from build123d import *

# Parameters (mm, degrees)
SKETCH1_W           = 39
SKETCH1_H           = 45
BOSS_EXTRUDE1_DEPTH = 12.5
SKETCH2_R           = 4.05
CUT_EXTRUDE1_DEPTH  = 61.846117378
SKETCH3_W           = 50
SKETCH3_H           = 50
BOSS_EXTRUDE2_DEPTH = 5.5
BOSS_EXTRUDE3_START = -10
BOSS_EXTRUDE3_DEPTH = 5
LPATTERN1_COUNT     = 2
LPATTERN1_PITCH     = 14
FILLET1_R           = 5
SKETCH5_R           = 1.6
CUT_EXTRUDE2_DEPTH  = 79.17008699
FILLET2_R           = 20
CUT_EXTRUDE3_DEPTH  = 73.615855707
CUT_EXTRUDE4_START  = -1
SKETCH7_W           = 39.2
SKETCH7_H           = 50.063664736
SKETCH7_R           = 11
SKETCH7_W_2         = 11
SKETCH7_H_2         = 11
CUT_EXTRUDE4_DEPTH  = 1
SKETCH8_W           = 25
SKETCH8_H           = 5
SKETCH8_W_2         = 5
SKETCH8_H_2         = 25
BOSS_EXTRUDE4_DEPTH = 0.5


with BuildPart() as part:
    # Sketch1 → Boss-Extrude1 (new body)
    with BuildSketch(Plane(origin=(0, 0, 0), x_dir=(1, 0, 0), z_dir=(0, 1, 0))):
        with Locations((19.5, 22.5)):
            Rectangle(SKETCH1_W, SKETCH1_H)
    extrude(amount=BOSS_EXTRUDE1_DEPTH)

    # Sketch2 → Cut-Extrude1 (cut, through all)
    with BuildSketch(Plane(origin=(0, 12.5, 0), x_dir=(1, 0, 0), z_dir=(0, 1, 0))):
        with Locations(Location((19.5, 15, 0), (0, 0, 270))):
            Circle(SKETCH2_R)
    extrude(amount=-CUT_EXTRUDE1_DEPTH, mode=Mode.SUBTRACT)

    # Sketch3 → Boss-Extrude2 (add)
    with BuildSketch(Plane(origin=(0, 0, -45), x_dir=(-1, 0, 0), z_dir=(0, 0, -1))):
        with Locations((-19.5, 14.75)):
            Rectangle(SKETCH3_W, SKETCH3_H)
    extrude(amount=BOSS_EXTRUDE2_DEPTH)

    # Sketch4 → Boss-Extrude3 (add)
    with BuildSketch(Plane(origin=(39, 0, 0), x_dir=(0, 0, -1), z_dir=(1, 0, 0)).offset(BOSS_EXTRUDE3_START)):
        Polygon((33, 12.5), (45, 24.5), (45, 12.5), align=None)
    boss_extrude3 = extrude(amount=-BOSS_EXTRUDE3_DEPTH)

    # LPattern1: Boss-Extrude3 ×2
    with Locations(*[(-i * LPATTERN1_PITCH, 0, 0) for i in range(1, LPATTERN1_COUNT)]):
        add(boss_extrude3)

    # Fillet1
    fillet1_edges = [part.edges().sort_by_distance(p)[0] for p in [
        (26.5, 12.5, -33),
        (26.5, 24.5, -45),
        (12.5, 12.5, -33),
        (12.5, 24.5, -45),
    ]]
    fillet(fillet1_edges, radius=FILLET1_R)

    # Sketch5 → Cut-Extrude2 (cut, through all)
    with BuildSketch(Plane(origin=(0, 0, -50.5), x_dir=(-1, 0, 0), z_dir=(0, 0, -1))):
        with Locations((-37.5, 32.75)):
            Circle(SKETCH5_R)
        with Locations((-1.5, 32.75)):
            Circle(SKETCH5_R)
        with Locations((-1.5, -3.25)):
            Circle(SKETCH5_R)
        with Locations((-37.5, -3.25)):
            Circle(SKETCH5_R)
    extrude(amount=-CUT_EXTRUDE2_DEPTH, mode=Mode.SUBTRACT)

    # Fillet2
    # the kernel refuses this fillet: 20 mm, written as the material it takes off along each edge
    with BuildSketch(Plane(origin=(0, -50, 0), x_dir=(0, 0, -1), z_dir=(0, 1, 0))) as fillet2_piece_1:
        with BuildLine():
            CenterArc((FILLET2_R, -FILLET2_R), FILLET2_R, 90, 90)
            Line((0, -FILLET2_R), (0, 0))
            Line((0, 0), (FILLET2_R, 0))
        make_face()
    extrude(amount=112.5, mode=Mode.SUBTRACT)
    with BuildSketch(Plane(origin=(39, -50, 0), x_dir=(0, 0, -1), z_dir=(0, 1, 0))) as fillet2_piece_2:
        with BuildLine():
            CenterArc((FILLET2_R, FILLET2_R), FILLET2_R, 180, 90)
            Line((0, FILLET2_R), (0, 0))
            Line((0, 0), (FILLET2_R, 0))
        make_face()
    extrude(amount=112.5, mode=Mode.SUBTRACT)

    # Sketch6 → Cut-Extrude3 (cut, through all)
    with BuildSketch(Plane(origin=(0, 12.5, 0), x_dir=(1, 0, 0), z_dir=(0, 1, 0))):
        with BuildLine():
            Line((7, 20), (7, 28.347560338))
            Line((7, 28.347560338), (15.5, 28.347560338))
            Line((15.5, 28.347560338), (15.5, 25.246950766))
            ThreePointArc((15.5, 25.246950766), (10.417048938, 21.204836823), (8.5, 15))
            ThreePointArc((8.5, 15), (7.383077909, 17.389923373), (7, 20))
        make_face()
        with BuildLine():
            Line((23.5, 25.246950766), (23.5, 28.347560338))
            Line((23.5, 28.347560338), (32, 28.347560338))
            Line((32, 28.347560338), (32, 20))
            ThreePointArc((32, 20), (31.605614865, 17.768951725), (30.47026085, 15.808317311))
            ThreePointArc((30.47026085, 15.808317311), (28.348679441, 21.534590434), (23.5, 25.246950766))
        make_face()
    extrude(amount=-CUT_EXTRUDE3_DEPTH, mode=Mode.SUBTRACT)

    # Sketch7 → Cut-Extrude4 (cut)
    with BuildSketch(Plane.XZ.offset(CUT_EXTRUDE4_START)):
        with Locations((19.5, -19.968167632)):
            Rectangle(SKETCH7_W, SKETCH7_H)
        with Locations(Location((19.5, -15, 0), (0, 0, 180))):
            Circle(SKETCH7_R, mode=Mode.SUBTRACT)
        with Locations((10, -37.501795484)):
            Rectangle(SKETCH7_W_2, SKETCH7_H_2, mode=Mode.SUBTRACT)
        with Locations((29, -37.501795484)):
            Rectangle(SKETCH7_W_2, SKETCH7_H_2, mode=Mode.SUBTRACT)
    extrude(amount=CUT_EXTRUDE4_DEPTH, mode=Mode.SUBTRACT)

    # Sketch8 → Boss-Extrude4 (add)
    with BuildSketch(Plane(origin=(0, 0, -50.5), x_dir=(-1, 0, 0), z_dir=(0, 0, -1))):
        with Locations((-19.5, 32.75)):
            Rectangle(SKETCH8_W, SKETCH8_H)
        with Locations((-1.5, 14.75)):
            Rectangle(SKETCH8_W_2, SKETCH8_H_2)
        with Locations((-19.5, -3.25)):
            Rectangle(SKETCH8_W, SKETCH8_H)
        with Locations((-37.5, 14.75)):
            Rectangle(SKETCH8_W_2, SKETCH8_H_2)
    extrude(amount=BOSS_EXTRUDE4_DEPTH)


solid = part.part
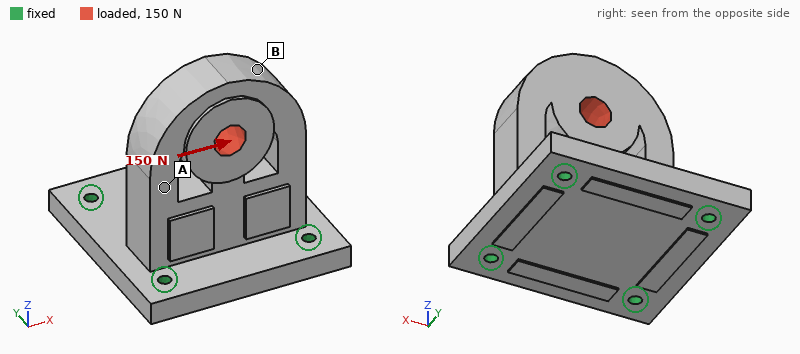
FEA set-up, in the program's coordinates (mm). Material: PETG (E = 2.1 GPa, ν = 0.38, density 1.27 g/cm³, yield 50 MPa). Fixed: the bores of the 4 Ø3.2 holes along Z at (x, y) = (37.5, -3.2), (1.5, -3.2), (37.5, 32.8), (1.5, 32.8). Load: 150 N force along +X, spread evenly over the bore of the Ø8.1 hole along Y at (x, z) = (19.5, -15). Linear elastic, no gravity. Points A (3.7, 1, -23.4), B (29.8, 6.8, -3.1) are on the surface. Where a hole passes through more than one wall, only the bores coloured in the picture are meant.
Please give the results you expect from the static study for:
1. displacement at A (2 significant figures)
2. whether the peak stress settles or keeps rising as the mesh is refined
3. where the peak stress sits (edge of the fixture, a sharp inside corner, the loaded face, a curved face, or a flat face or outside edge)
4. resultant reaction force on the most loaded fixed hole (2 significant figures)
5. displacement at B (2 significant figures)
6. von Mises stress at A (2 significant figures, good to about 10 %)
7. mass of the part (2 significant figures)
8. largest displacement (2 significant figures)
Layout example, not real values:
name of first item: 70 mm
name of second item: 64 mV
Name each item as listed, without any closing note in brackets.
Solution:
displacement at A: 0.076 mm
whether the peak stress settles or keeps rising as the mesh is refined: keeps rising
where the peak stress sits: edge of the fixture
resultant reaction force on the most loaded fixed hole: 130 N
displacement at B: 0.12 mm
von Mises stress at A: 1.2 MPa
mass of the part: 40 g
largest displacement: 0.13 mm
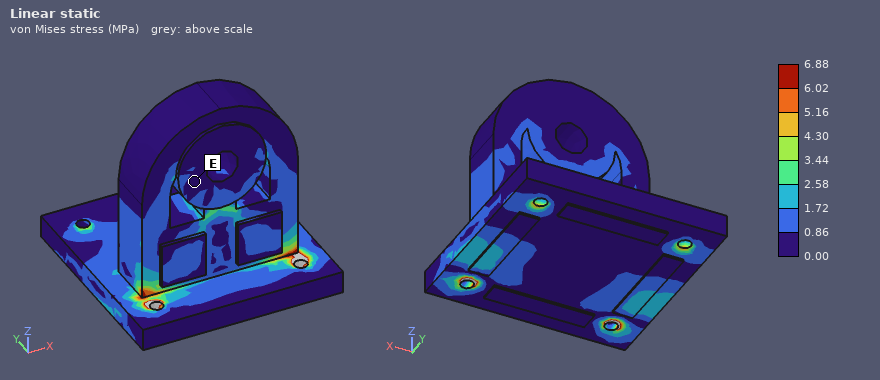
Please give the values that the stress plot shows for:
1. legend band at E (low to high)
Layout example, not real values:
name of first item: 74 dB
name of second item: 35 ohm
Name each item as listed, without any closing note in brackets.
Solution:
legend band at E: 0.00 to 0.86 MPa
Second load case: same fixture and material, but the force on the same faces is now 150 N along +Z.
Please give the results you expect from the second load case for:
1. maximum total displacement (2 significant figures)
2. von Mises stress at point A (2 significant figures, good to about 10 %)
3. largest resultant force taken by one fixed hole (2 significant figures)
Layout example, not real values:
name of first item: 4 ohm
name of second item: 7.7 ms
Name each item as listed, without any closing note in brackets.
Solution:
maximum total displacement: 28 µm
von Mises stress at point A: 0.54 MPa
largest resultant force taken by one fixed hole: 59 N
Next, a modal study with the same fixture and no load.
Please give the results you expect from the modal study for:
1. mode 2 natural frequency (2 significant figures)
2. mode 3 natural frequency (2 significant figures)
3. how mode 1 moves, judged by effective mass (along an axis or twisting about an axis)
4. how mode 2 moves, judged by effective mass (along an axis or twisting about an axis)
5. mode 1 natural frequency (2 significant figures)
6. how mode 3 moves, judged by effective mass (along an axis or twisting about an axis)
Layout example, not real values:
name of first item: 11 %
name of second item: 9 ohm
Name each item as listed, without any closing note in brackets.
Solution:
mode 2 natural frequency: 1700 Hz
mode 3 natural frequency: 2700 Hz
how mode 1 moves, judged by effective mass: along Y
how mode 2 moves, judged by effective mass: along X
mode 1 natural frequency: 1000 Hz
how mode 3 moves, judged by effective mass: along Z
